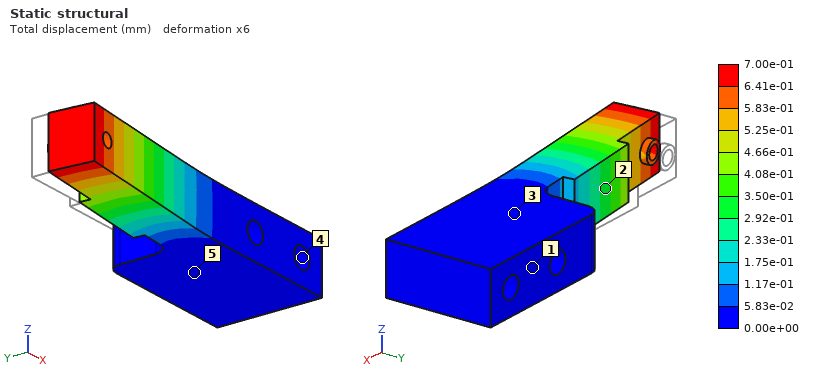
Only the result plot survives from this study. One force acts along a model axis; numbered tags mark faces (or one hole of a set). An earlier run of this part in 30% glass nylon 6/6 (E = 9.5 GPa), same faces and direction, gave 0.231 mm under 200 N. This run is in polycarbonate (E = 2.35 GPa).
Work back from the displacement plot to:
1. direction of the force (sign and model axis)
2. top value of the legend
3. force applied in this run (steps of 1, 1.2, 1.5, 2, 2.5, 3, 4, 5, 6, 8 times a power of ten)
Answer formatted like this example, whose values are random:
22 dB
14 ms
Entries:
-Y
7.00e-01 mm
150 N
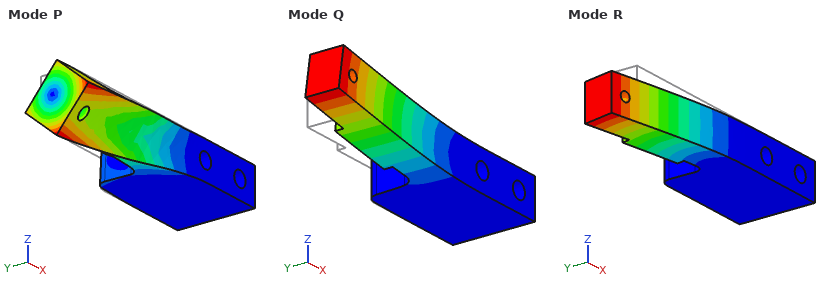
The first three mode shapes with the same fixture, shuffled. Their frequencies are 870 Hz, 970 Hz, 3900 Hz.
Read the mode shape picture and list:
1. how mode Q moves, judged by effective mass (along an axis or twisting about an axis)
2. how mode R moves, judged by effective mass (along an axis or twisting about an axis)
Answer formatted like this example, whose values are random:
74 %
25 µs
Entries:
along Z
along Y
